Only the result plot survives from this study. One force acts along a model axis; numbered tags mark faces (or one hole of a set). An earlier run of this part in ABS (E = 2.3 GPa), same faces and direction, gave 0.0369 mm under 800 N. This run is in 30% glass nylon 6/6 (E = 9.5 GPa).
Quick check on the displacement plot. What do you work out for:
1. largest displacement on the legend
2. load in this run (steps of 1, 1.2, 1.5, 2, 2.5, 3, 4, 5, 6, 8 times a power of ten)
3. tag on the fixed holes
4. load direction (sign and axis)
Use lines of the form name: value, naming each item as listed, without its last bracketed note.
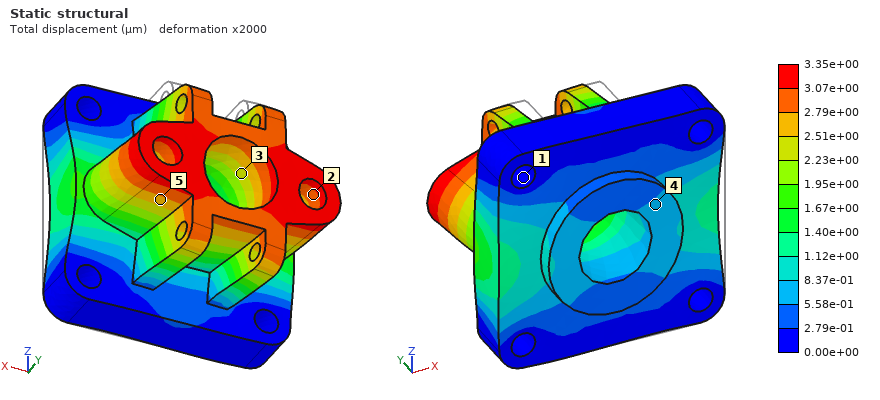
largest displacement on the legend: 3.35e+00 µm
load in this run: 300 N
tag on the fixed holes: 1
load direction: -X
